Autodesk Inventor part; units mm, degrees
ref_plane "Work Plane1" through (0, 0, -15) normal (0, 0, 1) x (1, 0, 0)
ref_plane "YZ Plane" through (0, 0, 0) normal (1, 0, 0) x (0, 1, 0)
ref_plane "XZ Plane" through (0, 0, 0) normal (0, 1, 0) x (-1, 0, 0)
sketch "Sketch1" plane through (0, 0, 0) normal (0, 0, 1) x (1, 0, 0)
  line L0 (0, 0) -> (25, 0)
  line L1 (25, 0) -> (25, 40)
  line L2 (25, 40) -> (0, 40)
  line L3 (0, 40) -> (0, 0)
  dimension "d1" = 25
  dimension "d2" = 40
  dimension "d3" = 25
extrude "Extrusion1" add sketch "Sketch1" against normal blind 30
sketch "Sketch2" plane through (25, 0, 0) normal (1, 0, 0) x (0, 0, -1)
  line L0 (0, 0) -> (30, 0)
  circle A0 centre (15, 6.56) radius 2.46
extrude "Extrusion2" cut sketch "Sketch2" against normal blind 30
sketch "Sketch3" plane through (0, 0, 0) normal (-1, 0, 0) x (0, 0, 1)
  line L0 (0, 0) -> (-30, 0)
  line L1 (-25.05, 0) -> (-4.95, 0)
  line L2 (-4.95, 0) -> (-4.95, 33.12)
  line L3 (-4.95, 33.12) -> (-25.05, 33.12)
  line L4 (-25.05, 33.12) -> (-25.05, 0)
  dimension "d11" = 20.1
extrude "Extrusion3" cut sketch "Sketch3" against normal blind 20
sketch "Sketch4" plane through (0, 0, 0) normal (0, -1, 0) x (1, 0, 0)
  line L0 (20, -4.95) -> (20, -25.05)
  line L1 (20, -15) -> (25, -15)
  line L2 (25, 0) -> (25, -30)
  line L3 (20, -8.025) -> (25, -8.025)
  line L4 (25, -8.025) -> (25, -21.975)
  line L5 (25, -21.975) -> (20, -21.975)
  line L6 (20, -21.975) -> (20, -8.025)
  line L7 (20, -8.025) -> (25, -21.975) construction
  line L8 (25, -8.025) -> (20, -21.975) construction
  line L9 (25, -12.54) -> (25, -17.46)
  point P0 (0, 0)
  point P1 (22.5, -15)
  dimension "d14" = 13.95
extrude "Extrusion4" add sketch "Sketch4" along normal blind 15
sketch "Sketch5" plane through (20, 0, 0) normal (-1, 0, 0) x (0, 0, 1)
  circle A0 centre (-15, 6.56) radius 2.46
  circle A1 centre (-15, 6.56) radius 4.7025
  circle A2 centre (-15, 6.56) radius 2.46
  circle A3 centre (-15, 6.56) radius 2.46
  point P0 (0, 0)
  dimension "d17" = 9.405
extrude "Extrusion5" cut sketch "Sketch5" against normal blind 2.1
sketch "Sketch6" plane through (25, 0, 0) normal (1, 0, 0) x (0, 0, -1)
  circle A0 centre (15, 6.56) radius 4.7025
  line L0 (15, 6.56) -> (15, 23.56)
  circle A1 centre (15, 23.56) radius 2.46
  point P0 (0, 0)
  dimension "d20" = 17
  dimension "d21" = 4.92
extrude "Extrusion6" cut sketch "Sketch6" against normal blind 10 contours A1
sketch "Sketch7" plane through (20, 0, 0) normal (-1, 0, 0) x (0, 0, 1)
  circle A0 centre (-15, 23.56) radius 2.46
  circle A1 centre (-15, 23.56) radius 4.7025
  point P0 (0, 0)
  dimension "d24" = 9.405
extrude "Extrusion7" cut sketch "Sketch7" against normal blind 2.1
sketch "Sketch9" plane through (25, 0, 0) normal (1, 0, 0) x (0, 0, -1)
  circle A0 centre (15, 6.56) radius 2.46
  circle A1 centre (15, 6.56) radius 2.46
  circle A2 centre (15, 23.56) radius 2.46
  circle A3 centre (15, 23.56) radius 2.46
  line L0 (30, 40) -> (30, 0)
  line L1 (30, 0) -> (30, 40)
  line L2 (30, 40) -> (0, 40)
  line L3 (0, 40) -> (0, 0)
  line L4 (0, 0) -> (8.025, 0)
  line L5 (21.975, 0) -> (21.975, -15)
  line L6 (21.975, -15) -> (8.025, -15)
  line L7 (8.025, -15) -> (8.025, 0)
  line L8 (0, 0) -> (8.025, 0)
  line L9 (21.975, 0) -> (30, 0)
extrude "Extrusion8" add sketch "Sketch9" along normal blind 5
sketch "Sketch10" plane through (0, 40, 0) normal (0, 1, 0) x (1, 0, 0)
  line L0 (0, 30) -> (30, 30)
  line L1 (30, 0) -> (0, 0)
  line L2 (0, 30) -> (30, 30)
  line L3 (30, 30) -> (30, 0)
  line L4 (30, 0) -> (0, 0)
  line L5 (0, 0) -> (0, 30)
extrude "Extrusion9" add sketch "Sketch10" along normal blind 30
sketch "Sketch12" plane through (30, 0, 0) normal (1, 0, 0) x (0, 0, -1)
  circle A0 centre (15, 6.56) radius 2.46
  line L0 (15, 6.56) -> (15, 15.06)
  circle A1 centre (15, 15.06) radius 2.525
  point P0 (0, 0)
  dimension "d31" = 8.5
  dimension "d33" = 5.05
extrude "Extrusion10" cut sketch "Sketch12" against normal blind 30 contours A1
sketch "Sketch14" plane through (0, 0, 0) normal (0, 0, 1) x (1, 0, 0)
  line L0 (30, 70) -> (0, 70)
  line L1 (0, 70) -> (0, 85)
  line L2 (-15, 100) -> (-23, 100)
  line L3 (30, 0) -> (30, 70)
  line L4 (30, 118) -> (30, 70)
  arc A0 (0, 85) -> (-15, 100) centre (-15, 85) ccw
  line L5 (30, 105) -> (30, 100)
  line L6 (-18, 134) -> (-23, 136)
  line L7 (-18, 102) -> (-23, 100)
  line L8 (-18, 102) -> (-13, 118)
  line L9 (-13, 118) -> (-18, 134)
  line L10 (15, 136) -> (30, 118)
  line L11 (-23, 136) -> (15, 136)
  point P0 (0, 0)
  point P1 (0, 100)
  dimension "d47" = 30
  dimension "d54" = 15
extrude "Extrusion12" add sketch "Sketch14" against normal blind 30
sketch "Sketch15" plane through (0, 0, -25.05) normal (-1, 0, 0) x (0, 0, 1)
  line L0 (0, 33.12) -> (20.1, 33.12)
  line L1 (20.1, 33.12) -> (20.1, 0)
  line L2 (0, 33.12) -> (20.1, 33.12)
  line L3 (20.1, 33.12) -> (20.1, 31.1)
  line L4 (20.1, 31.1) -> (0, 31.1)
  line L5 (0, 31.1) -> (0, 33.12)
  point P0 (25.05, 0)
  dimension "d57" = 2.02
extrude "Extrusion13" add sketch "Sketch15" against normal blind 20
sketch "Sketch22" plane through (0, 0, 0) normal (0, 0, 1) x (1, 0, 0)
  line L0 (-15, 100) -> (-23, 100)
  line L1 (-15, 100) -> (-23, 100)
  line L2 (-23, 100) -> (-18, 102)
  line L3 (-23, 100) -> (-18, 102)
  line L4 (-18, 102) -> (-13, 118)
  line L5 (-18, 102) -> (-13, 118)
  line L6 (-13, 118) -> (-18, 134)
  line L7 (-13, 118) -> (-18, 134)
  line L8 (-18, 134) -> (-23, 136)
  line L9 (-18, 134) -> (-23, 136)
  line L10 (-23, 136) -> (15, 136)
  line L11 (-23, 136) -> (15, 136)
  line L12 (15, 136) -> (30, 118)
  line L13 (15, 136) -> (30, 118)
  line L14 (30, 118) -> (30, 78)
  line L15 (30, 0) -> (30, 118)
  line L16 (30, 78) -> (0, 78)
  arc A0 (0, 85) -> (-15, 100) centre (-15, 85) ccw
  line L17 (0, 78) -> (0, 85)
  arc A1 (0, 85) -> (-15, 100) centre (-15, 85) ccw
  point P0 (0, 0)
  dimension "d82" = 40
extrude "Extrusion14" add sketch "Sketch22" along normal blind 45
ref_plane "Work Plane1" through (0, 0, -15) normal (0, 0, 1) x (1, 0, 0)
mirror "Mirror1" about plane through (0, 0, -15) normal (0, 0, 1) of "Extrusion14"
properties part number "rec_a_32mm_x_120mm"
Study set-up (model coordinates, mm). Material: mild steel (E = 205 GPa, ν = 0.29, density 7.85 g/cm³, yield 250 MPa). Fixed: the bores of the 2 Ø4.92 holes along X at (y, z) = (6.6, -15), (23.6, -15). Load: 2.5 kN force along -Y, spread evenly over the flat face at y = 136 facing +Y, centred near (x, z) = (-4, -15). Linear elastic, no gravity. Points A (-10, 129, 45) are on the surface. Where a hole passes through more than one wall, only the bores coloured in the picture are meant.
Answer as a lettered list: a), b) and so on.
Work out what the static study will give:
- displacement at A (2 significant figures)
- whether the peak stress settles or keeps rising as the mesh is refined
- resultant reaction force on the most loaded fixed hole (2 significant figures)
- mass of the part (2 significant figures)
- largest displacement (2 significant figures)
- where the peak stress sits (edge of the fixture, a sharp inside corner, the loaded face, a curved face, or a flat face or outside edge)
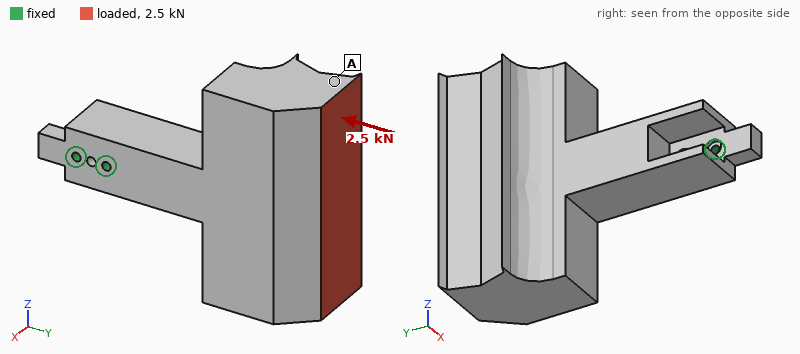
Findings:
a) 75 µm
b) keeps rising
c) 3.4 kN
d) 2.6 kg
e) 85 µm
f) edge of the fixture
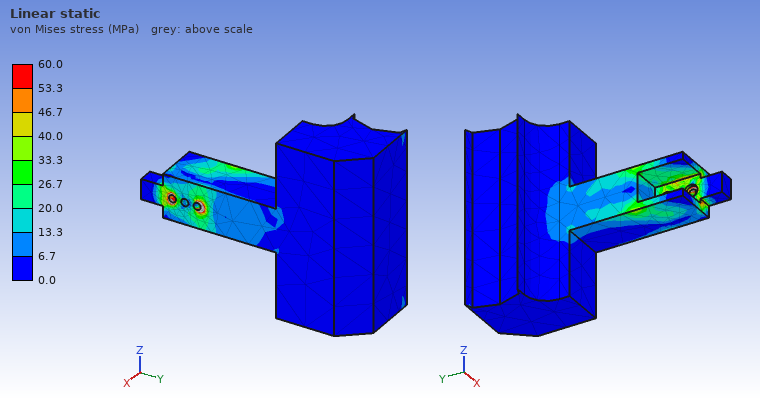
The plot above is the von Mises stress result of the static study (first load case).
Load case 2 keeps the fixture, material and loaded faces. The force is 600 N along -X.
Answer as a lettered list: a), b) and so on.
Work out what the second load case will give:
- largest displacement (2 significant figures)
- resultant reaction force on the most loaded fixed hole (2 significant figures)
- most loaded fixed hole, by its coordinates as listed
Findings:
a) 79 µm
b) 3.3 kN
c) (23.6, -15)
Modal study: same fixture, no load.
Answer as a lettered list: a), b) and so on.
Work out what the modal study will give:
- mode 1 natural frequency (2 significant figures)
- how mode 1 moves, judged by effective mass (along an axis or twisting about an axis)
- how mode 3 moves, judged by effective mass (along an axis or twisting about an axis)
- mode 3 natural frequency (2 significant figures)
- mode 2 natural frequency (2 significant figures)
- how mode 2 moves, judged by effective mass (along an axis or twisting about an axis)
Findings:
a) 400 Hz
b) along X
c) twisting about Y
d) 640 Hz
e) 440 Hz
f) along Z
